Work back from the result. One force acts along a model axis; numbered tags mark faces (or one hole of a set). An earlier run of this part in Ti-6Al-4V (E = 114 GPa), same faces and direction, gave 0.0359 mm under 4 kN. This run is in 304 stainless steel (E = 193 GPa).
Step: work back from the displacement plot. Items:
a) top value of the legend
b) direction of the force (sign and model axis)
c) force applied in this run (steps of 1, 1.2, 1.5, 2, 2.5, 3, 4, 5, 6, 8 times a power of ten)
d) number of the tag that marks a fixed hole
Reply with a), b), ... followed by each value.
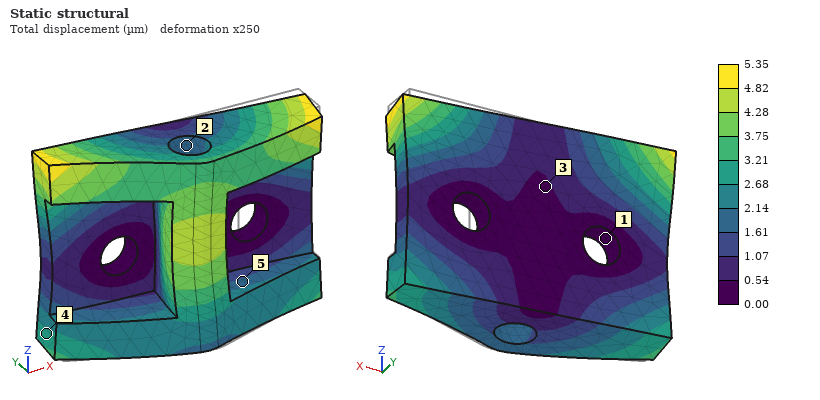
a) 5.35 µm
b) -X
c) 1 kN
d) 1
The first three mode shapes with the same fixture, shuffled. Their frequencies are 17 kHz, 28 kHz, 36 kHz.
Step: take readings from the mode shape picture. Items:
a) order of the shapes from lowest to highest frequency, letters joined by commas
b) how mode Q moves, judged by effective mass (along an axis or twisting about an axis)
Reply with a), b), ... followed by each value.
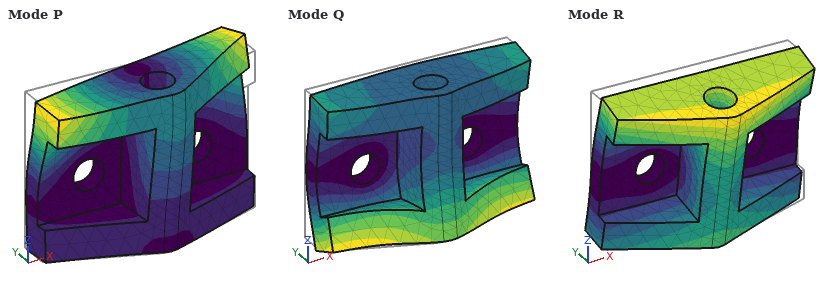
a) R, P, Q
b) along Y
